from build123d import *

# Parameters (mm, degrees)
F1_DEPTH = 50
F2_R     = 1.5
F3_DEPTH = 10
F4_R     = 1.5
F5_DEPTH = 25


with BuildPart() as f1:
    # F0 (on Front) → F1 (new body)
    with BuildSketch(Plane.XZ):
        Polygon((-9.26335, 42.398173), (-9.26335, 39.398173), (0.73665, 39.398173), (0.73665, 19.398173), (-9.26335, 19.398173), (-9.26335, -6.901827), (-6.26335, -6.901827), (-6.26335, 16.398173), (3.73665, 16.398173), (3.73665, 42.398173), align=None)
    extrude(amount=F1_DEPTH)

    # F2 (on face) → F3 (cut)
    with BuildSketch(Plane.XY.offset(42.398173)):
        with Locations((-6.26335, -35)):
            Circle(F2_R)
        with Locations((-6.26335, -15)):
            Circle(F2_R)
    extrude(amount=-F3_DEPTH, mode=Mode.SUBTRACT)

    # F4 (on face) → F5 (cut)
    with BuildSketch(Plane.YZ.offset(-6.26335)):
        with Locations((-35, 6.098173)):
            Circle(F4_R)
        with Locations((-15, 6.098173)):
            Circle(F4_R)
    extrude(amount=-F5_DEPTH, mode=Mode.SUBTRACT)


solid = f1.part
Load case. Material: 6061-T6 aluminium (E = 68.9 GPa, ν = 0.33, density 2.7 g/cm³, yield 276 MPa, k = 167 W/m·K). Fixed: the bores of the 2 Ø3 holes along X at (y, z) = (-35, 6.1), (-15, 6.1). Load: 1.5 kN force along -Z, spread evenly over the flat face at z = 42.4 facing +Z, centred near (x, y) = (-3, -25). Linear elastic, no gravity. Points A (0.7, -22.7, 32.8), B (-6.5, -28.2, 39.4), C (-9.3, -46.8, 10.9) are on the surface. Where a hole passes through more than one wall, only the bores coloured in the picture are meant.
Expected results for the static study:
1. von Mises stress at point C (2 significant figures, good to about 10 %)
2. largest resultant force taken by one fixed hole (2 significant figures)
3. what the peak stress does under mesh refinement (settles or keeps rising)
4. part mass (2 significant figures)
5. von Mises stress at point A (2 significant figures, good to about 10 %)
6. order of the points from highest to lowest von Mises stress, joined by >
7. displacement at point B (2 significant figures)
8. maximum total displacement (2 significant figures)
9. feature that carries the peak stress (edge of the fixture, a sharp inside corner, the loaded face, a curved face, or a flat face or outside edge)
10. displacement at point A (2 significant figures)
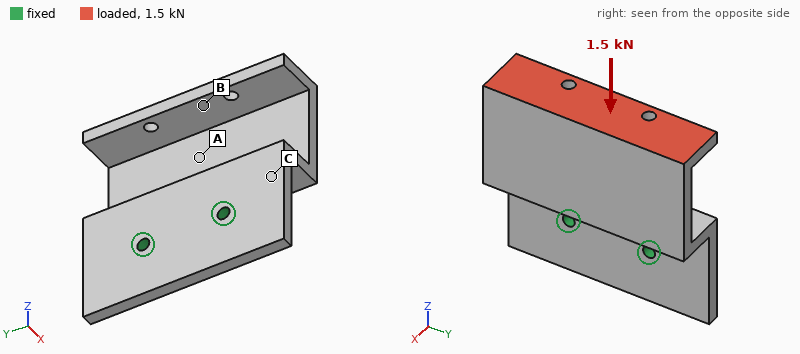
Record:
69 MPa
750 N
keeps rising
28 g
97 MPa
A > C > B
0.26 mm
0.29 mm
edge of the fixture
0.22 mm
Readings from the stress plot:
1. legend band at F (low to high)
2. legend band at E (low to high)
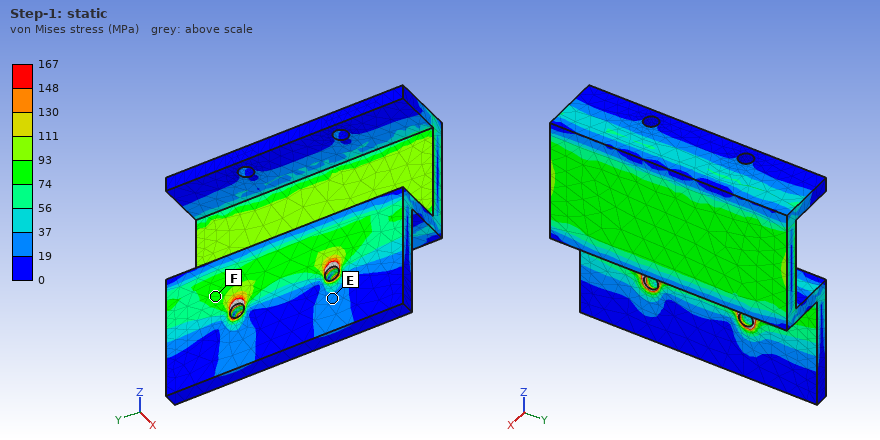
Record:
74 to 93 MPa
19 to 37 MPa
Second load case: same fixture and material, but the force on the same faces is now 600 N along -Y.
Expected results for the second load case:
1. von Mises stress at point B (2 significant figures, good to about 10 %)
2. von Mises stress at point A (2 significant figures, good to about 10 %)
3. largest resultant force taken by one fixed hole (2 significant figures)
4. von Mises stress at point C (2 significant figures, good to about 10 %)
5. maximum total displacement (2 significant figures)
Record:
20 MPa
43 MPa
1.0 kN
37 MPa
0.29 mm
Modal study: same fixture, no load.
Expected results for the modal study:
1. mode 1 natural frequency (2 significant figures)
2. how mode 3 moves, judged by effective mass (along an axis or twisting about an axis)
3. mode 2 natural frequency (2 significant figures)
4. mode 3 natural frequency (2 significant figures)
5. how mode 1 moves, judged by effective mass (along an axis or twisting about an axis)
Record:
1100 Hz
along Z
2300 Hz
4500 Hz
along X
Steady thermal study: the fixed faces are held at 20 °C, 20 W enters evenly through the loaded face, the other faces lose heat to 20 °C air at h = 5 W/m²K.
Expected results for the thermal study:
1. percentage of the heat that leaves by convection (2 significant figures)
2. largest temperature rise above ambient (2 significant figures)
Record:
3.1 %
39 K
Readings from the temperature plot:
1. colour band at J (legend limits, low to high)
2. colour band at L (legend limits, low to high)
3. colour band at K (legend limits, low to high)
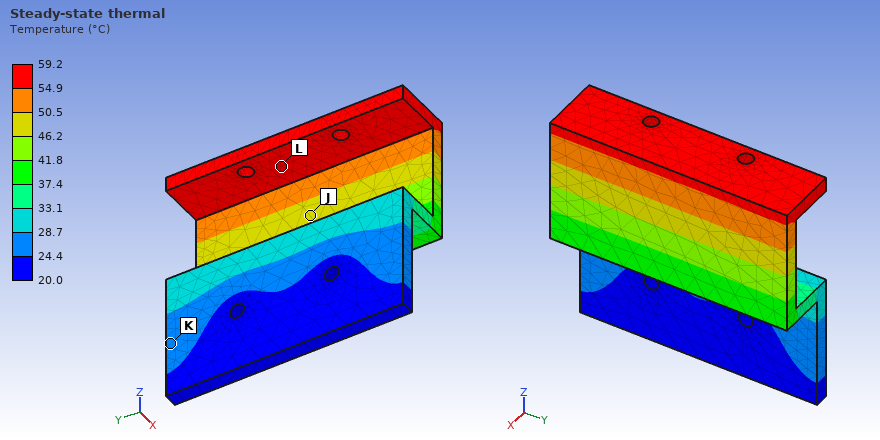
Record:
46.2 to 50.5 °C
54.9 to 59.2 °C
24.4 to 28.7 °C
